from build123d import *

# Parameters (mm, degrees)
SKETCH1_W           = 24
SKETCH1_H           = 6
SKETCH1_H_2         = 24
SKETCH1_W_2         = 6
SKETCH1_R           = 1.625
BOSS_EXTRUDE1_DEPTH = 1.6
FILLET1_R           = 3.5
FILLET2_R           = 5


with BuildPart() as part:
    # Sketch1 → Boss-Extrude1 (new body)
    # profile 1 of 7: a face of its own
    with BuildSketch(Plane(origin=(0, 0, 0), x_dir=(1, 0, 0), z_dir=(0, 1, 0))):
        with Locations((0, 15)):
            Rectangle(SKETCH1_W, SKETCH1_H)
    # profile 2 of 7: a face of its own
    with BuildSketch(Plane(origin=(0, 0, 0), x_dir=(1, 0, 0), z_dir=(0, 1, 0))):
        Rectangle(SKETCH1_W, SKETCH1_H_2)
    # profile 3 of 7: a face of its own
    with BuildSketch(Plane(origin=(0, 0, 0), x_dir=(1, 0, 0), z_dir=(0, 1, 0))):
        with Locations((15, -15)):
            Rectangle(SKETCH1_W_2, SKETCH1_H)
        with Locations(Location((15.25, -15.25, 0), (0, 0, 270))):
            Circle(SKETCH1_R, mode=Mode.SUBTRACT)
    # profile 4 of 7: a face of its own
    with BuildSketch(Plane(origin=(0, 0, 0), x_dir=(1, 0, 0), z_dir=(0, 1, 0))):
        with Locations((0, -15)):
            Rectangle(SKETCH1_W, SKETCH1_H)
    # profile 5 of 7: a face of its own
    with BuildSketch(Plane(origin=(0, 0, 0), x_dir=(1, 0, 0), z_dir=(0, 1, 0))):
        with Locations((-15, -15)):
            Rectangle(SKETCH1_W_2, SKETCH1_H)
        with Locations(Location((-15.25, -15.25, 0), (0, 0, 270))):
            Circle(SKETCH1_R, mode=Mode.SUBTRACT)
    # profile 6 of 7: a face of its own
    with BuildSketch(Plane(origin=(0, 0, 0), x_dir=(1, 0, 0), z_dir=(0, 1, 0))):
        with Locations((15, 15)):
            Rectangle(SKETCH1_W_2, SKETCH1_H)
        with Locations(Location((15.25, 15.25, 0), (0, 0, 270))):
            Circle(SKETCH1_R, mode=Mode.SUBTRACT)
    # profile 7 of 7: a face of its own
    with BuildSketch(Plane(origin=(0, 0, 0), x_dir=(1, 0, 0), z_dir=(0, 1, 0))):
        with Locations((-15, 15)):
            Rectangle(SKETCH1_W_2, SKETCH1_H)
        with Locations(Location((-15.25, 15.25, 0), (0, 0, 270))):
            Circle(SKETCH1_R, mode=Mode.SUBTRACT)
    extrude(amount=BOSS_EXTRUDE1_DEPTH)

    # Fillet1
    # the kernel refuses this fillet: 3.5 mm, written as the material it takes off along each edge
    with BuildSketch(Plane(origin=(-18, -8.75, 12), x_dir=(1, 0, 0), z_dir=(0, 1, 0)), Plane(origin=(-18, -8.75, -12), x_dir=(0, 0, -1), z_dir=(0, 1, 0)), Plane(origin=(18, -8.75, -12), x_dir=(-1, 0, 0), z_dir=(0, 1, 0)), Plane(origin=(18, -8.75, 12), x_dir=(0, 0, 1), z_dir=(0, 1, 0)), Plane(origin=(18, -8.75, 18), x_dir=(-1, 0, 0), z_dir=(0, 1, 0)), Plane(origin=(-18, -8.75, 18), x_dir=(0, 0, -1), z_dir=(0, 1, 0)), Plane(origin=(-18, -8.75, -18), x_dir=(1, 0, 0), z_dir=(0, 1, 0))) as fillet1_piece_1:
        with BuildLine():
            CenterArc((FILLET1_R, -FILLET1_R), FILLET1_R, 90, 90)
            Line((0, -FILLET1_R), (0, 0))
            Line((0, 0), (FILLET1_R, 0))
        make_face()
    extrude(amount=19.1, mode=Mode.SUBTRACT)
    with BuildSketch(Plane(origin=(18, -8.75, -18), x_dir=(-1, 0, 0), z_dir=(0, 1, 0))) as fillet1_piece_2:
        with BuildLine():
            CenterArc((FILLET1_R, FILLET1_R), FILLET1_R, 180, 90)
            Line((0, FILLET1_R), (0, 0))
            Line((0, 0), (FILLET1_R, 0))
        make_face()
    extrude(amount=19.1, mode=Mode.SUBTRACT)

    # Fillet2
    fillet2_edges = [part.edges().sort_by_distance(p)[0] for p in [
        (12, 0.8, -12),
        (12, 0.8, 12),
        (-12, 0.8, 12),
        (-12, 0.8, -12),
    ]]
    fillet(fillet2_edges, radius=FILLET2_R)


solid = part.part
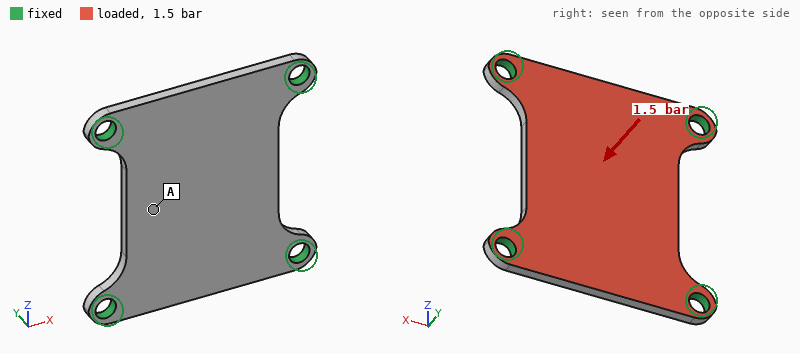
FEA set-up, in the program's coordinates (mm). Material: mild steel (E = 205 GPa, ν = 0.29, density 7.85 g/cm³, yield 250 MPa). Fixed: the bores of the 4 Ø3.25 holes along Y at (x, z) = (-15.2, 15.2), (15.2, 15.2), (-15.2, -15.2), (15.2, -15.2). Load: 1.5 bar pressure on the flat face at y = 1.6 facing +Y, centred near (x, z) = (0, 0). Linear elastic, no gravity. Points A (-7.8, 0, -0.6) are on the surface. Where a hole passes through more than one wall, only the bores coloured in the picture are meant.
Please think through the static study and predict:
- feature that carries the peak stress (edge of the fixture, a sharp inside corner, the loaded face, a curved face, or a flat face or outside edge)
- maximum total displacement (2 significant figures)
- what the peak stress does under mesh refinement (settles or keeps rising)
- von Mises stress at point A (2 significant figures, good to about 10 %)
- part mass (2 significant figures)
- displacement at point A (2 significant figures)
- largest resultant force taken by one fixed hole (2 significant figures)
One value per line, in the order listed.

edge of the fixture
12 µm
keeps rising
16 MPa
12 g
9.8 µm
36 N
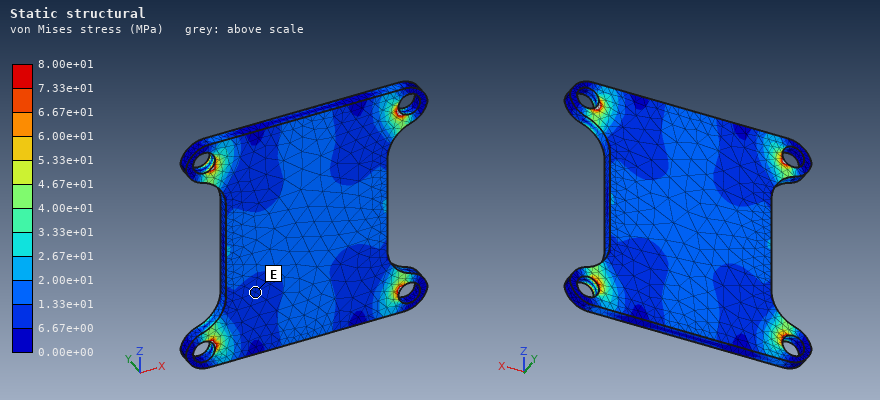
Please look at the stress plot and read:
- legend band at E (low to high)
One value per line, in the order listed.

6.67e+00 to 1.33e+01 MPa
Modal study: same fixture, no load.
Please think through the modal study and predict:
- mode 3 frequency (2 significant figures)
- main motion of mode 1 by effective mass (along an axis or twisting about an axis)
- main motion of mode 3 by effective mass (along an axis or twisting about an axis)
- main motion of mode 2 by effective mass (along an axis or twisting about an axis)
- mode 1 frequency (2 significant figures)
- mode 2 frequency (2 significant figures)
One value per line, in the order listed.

12 kHz
along Y
twisting about Z
twisting about X
6100 Hz
11 kHz
